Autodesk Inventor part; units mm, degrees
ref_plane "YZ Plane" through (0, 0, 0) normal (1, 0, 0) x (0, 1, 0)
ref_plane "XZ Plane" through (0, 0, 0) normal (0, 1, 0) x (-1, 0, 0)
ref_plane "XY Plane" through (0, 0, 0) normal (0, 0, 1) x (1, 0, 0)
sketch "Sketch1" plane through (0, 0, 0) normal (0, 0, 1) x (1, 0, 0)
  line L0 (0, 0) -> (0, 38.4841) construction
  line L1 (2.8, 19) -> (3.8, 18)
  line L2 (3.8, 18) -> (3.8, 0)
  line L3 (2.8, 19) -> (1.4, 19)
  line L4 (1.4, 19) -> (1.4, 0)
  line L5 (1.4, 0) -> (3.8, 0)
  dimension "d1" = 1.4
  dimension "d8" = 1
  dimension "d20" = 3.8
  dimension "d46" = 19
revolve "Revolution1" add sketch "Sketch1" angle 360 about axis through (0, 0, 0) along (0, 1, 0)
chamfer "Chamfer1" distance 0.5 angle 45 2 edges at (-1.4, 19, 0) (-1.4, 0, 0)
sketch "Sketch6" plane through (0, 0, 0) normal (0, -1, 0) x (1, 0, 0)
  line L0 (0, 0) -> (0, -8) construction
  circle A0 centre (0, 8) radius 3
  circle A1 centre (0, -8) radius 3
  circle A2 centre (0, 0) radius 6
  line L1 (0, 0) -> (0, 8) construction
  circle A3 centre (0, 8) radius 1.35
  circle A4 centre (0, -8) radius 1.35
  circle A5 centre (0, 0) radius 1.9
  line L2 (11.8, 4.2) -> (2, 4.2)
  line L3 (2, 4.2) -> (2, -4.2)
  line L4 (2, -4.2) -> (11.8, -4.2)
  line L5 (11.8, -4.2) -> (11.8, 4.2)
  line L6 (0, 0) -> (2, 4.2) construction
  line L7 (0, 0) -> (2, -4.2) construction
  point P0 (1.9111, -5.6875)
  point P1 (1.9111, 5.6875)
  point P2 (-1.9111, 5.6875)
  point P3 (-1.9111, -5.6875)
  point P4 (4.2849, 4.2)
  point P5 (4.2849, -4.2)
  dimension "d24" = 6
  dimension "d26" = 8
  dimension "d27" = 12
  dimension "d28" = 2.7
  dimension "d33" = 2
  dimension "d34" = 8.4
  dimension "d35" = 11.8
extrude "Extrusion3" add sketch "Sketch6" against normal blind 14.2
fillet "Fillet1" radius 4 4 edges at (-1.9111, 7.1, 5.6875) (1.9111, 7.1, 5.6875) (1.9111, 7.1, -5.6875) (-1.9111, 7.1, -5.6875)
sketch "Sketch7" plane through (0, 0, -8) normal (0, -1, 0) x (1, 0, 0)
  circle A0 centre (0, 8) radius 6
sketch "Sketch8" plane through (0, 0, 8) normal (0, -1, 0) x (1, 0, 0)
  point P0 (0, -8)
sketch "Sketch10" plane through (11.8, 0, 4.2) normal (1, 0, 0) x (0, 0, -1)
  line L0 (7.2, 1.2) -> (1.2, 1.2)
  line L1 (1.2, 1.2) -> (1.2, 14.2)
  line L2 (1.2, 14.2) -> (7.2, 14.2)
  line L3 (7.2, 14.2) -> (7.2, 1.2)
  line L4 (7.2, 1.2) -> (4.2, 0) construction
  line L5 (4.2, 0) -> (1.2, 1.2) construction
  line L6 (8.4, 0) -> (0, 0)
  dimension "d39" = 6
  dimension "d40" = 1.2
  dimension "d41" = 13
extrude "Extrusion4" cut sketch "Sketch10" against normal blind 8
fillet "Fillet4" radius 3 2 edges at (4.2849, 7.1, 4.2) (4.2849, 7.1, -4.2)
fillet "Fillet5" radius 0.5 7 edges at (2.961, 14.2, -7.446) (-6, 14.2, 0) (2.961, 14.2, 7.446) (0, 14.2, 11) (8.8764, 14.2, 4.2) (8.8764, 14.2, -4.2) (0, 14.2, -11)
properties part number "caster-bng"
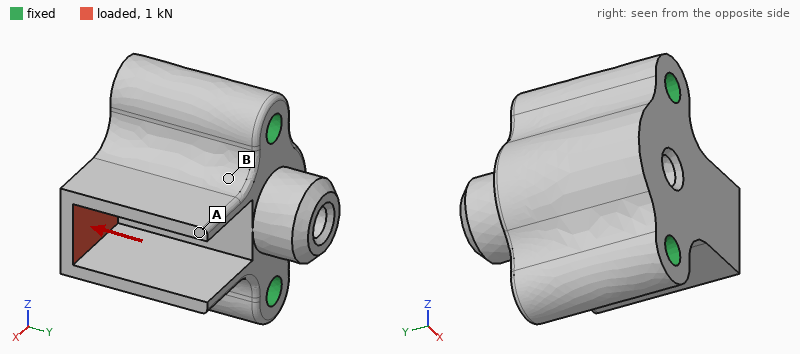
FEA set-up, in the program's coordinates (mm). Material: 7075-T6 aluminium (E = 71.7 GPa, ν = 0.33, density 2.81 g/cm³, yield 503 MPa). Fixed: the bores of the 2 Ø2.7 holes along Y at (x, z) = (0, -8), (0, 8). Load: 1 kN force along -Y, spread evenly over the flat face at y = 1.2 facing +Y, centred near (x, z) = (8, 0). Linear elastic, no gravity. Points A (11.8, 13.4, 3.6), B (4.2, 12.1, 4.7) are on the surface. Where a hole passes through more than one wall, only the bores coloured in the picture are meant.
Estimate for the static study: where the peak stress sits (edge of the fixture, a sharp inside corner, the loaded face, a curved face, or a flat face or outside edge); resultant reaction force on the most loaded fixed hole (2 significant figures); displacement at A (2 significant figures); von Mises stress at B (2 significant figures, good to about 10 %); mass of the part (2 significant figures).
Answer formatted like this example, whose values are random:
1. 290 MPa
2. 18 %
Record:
1. a flat face or outside edge
2. 500 N
3. 15 µm
4. 45 MPa
5. 7.0 g
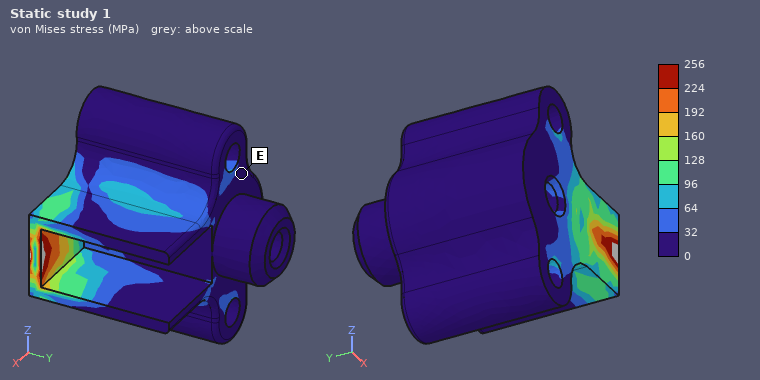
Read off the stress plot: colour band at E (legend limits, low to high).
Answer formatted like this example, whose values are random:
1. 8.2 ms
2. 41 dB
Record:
1. 0 to 32 MPa
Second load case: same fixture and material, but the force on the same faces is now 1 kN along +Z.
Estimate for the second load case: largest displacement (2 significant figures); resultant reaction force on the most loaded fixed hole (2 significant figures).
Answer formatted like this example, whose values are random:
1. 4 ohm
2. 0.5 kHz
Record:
1. 30 µm
2. 730 N
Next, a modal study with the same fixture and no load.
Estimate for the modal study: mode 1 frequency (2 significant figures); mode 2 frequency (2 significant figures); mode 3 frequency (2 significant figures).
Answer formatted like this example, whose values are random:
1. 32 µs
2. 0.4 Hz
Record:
1. 21 kHz
2. 21 kHz
3. 42 kHz
